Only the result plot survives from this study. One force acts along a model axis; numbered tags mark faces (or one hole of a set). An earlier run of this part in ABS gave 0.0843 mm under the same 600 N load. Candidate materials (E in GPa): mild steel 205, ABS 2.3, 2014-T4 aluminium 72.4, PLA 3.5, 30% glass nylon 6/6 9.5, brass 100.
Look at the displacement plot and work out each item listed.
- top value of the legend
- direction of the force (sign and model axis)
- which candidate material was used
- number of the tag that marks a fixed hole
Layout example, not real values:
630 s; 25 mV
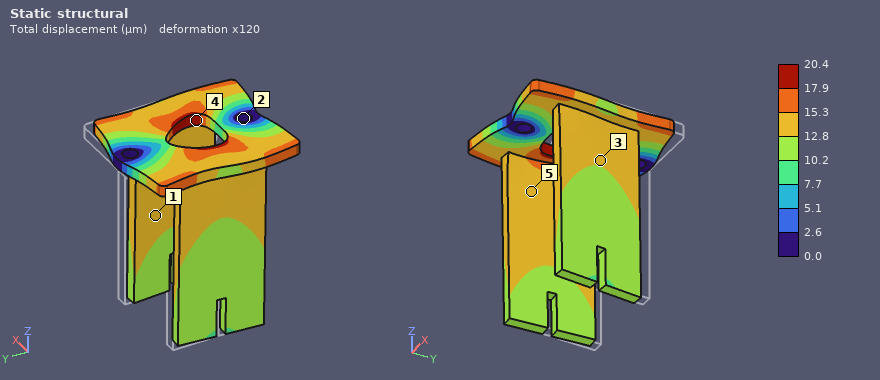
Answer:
20.4 µm; -Y; 30% glass nylon 6/6; 2
